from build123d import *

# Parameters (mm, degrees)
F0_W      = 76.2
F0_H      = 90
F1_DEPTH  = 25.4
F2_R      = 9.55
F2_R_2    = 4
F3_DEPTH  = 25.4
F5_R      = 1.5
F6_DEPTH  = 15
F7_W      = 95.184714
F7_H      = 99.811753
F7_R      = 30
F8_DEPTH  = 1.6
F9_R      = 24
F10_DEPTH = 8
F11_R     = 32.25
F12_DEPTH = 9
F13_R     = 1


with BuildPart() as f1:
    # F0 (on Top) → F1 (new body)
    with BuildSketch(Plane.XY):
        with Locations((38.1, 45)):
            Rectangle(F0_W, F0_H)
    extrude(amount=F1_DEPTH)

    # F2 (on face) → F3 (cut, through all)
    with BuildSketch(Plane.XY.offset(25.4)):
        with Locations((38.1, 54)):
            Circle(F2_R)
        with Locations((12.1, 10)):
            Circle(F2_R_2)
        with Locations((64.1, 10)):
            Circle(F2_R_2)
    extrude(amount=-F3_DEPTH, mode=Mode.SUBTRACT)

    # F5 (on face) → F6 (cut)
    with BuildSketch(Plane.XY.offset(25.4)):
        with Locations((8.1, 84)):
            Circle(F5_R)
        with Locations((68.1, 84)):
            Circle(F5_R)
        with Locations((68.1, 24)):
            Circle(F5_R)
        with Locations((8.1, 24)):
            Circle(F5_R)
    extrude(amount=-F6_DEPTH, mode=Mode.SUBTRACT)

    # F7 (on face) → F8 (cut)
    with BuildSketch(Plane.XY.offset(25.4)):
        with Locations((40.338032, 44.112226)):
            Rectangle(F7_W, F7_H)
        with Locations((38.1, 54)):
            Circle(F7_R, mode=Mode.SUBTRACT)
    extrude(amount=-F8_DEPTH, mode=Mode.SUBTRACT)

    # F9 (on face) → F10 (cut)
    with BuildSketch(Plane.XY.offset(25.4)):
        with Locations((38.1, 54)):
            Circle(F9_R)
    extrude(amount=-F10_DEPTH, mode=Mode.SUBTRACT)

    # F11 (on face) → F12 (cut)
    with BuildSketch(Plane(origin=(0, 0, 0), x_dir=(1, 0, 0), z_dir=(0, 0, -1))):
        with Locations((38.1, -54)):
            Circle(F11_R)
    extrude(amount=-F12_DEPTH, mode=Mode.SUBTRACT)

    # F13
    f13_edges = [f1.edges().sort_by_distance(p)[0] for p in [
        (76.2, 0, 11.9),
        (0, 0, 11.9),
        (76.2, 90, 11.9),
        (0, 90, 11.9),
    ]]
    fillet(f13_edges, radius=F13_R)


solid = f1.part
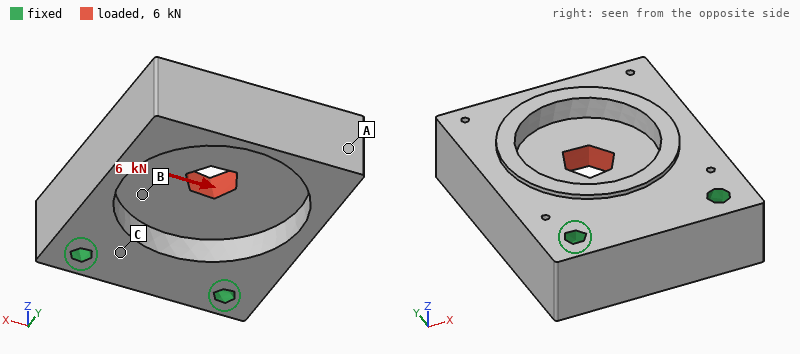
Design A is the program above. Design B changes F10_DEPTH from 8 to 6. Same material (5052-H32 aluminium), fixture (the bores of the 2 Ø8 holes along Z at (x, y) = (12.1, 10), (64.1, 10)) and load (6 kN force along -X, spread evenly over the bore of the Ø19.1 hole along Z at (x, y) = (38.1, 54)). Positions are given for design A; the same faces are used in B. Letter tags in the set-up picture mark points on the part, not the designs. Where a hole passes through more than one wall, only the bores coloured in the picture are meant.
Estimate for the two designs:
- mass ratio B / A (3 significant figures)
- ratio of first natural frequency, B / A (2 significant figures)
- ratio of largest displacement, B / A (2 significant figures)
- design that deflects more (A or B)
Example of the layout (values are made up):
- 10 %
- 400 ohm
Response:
- 1.03
- 1.0
- 0.92
- A
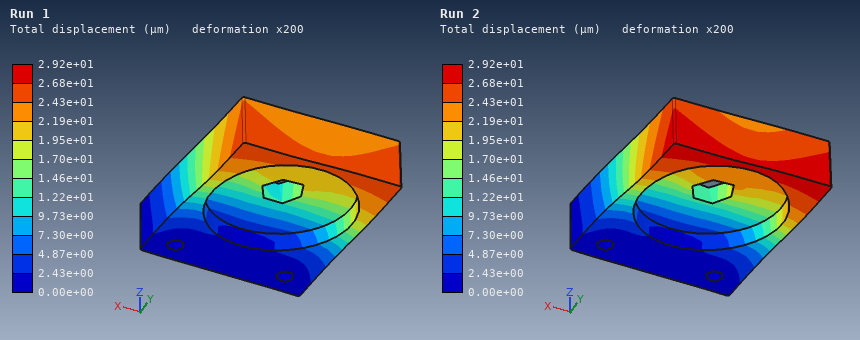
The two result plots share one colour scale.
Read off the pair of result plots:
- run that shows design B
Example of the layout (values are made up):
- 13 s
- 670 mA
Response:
- Run 1
